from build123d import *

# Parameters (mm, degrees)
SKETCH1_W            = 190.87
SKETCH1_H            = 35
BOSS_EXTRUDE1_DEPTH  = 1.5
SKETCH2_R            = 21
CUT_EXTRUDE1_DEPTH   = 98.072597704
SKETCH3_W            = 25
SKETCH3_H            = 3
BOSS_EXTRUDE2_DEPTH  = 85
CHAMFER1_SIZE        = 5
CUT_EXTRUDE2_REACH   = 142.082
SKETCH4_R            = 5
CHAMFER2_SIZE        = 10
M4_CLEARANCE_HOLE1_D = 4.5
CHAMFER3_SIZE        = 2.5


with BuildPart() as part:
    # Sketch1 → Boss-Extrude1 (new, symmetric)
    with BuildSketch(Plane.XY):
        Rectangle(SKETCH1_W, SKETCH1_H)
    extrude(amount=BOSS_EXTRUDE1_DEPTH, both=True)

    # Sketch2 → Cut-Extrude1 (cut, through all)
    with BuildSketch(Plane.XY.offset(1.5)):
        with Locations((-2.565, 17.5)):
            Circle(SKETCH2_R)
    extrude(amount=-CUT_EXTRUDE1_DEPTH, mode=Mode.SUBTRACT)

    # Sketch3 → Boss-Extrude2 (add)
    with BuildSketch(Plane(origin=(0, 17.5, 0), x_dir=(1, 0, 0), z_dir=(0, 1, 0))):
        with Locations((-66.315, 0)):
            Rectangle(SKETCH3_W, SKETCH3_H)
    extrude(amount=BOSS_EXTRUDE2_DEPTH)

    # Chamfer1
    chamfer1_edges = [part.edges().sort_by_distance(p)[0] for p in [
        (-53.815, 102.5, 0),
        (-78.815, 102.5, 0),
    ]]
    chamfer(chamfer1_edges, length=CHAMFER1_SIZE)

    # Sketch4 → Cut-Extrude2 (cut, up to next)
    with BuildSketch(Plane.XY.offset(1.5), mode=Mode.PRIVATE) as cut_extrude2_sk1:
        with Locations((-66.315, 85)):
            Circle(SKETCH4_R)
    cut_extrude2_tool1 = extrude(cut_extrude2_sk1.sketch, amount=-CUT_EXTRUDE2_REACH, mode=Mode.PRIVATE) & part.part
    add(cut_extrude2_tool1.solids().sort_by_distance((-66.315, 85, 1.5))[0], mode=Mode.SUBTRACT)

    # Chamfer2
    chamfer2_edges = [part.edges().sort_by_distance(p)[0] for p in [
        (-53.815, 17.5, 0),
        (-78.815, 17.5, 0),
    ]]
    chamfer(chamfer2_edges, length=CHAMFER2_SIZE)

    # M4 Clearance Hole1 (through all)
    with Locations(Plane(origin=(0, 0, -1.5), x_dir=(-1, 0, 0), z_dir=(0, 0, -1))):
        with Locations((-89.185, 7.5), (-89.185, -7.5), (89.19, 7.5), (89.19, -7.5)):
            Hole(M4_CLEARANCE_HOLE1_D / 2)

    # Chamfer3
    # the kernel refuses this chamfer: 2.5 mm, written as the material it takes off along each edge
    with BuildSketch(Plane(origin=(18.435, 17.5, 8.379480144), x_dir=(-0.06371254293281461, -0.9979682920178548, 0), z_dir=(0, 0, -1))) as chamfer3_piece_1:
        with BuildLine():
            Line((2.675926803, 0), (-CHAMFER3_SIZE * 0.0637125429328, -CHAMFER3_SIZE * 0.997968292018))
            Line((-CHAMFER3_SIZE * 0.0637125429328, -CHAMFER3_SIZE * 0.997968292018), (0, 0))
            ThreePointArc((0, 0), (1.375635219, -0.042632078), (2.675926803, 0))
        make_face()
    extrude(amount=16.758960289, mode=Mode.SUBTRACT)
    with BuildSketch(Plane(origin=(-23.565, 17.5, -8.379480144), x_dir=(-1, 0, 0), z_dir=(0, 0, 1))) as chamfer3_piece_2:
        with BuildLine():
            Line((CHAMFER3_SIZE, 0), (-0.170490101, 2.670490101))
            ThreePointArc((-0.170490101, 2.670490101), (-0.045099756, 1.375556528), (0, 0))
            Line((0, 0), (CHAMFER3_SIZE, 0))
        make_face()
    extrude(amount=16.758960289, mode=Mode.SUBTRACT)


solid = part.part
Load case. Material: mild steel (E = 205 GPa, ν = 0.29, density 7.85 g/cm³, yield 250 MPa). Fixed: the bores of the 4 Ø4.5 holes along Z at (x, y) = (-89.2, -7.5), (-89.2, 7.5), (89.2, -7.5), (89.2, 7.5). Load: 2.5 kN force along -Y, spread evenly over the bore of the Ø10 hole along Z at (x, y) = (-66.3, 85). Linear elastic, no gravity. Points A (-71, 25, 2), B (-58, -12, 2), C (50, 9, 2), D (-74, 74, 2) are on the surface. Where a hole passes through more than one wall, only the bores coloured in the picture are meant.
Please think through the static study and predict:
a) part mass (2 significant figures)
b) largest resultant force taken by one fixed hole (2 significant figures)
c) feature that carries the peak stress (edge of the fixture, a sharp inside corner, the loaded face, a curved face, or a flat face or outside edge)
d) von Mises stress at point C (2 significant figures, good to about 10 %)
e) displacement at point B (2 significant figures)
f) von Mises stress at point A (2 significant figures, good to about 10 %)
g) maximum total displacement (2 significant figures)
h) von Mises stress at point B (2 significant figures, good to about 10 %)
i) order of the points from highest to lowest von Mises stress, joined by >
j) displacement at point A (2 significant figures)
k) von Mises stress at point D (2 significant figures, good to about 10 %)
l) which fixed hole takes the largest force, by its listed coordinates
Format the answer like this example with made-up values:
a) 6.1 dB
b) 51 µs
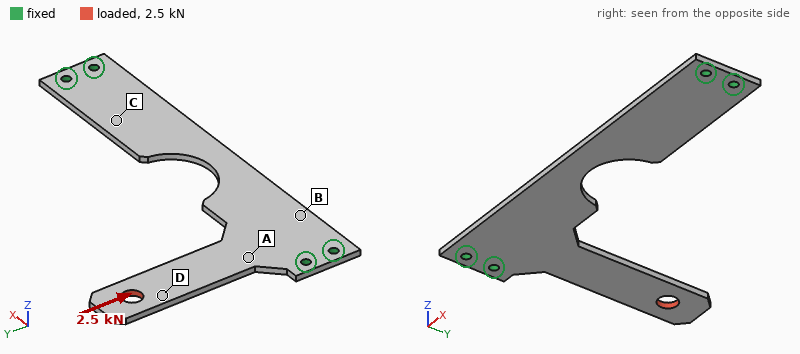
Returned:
a) 190 g
b) 2.3 kN
c) edge of the fixture
d) 8.2 MPa
e) 15 µm
f) 25 MPa
g) 51 µm
h) 14 MPa
i) D > A > B > C
j) 16 µm
k) 36 MPa
l) (-89.2, 7.5)
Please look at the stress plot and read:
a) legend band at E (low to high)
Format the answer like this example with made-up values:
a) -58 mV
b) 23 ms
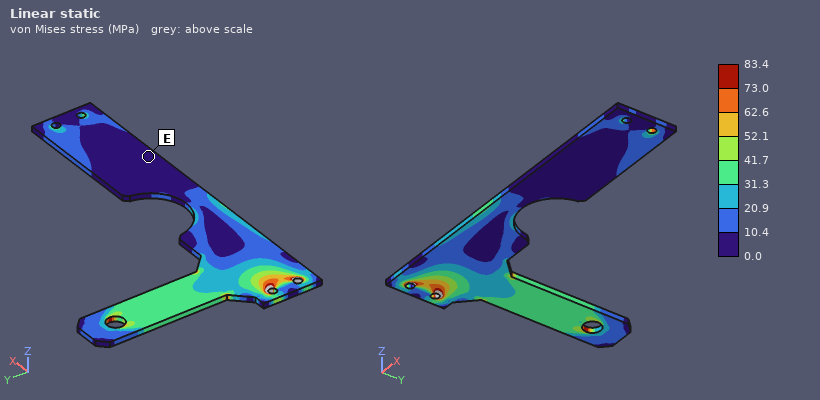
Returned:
a) 0.0 to 10.4 MPa
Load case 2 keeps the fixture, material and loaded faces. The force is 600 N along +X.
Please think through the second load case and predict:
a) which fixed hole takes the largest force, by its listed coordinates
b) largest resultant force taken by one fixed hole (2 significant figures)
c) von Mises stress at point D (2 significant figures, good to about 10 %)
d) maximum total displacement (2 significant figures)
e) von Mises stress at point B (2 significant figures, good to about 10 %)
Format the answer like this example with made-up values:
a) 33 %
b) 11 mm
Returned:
a) (-89.2, 7.5)
b) 2.1 kN
c) 15 MPa
d) 0.15 mm
e) 13 MPa
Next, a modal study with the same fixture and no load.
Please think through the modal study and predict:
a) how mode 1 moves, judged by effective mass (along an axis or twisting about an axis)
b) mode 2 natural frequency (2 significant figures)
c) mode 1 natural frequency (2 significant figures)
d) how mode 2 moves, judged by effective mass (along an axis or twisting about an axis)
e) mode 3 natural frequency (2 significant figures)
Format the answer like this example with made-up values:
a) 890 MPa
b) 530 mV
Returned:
a) along Z
b) 540 Hz
c) 290 Hz
d) along Z
e) 1200 Hz
